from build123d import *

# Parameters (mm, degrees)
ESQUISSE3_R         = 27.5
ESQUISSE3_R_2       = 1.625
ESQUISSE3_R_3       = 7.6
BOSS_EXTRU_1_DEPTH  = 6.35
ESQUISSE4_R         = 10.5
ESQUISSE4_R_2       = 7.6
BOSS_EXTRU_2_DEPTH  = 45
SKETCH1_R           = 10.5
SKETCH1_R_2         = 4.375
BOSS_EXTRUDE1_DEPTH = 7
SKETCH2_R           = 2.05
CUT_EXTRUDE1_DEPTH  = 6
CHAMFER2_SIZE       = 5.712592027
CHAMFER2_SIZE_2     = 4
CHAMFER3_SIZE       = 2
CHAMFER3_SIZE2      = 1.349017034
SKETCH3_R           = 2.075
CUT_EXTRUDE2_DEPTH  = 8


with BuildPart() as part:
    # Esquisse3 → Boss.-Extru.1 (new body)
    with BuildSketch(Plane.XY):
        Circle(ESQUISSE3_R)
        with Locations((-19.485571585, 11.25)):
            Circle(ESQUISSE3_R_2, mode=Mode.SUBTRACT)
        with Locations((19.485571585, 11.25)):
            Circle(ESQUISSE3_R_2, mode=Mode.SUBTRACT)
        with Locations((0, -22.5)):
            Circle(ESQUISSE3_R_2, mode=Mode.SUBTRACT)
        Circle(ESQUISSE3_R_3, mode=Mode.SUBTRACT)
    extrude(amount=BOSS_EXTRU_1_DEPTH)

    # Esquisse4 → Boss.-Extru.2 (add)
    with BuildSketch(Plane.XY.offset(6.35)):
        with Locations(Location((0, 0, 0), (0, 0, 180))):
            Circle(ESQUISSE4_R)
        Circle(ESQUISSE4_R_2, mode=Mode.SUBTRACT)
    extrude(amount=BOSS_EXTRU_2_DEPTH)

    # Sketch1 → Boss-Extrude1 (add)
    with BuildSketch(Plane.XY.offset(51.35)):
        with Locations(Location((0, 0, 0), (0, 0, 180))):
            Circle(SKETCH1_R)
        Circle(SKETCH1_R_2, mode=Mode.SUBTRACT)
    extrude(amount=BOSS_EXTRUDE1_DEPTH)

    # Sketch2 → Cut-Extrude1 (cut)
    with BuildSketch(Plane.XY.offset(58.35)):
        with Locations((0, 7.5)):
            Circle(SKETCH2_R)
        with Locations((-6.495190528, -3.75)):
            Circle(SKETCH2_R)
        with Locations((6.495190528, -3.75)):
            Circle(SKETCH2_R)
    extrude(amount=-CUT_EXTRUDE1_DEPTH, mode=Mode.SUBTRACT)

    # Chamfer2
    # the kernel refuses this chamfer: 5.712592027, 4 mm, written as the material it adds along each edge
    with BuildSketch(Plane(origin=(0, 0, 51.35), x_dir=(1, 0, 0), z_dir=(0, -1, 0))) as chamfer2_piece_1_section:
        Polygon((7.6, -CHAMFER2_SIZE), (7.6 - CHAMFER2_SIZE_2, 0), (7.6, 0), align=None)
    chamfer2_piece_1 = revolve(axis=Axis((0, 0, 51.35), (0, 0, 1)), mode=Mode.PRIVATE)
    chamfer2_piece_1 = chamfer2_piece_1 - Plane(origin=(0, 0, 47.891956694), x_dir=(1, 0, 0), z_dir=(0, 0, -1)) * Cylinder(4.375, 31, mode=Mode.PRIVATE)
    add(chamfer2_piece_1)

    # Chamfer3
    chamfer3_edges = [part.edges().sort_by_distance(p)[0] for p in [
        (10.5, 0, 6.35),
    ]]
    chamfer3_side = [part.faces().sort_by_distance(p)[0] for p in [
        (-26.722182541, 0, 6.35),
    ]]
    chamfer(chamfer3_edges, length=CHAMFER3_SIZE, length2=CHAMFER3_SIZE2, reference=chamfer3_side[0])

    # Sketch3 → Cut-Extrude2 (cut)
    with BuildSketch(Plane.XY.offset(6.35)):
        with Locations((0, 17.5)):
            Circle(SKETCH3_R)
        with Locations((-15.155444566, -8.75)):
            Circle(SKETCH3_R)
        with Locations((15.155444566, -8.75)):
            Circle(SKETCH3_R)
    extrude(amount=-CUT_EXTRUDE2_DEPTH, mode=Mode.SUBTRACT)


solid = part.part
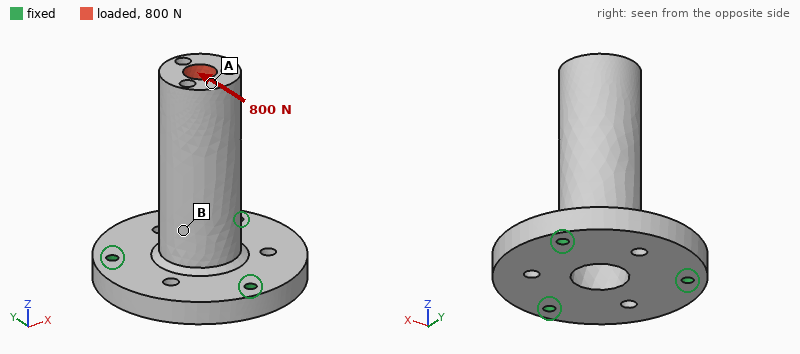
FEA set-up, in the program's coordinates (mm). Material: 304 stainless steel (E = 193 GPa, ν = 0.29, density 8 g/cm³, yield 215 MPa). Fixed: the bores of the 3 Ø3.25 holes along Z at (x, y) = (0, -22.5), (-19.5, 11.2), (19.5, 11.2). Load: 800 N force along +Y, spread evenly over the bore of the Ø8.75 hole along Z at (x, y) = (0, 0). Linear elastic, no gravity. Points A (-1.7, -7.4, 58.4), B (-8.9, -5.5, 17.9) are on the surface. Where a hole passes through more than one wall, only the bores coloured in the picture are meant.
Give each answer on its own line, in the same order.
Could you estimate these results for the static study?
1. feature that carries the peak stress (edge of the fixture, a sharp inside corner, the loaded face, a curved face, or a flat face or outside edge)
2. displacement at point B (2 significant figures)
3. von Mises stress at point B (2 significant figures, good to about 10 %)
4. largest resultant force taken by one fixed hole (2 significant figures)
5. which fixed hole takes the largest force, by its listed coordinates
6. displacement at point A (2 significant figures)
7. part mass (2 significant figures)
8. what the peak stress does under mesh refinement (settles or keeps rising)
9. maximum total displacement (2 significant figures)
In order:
edge of the fixture
11 µm
24 MPa
1.3 kN
(0, -22.5)
61 µm
190 g
keeps rising
62 µm
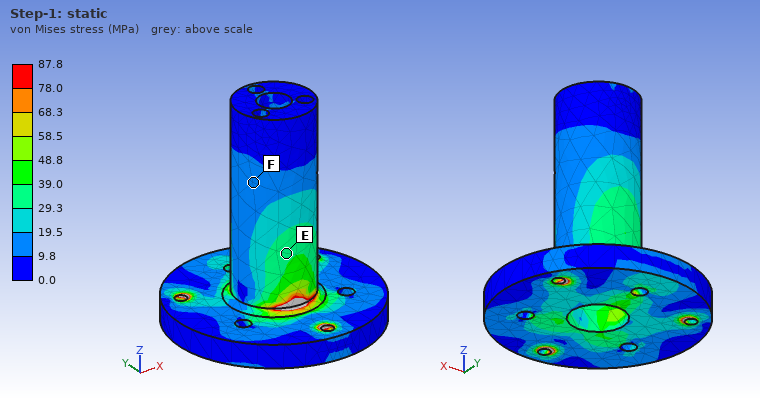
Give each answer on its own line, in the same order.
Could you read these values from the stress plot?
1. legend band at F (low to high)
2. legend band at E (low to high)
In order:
9.8 to 19.5 MPa
29.3 to 39.0 MPa
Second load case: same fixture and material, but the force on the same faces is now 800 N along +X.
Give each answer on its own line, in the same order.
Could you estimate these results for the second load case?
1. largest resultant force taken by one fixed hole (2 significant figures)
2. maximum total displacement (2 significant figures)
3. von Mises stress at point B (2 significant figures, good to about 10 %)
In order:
1.1 kN
62 µm
34 MPa
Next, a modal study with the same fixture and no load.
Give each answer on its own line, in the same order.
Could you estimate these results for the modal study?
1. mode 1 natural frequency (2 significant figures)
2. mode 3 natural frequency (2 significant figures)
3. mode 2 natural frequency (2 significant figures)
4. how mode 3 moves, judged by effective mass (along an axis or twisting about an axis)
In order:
3300 Hz
9700 Hz
3300 Hz
along Z
